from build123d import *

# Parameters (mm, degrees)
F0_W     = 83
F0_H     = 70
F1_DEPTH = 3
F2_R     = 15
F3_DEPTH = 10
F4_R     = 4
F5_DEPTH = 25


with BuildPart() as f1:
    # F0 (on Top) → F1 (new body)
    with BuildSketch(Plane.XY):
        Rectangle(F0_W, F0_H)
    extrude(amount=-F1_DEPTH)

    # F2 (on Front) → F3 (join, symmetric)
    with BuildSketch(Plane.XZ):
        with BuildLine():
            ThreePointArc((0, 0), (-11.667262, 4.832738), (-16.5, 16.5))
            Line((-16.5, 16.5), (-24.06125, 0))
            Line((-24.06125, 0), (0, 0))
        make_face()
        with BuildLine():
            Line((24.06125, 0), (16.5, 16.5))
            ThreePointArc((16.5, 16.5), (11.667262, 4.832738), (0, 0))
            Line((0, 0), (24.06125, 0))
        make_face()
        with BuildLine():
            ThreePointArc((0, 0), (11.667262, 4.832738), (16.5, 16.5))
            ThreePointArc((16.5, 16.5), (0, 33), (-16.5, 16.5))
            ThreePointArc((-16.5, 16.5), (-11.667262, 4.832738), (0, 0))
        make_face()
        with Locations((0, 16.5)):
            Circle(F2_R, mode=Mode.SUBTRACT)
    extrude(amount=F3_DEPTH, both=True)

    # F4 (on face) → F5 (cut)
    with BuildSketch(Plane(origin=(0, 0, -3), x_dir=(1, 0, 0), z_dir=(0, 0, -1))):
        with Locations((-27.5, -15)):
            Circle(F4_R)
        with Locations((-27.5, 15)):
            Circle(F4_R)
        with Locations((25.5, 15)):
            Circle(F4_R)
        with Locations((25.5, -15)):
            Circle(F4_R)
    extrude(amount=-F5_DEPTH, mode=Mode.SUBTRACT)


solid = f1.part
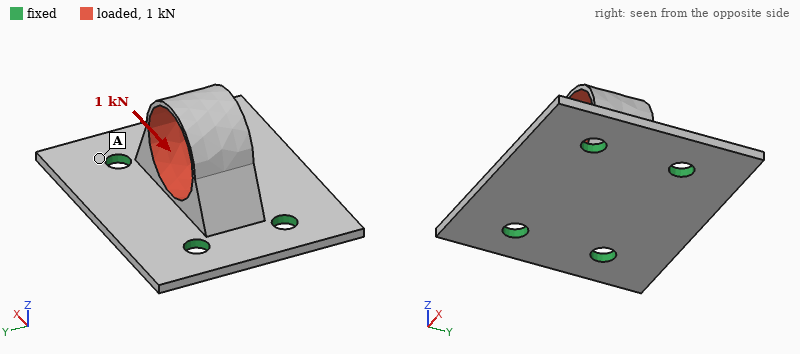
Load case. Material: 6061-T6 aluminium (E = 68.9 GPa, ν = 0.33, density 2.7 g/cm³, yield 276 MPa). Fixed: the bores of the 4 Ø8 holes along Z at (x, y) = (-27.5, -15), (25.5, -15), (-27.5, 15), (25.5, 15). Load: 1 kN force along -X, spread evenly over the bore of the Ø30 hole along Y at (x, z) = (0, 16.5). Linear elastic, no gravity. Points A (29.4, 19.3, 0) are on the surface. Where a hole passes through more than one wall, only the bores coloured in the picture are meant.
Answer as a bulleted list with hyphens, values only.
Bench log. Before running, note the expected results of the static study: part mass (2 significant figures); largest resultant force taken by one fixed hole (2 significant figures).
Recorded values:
- 66 g
- 340 N
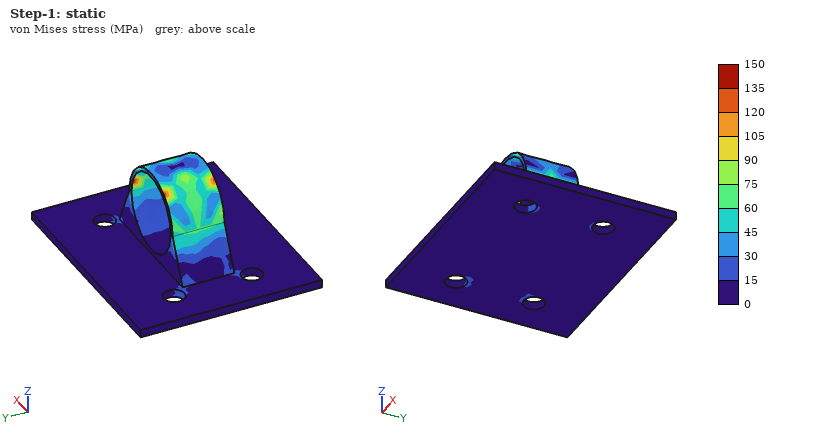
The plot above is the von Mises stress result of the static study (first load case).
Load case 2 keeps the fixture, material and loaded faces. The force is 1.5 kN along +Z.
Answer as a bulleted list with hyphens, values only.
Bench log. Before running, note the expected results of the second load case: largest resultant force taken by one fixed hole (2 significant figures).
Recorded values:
- 470 N
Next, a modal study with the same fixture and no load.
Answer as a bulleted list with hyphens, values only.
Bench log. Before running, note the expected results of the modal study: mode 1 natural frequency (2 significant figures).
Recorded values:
- 5400 Hz
